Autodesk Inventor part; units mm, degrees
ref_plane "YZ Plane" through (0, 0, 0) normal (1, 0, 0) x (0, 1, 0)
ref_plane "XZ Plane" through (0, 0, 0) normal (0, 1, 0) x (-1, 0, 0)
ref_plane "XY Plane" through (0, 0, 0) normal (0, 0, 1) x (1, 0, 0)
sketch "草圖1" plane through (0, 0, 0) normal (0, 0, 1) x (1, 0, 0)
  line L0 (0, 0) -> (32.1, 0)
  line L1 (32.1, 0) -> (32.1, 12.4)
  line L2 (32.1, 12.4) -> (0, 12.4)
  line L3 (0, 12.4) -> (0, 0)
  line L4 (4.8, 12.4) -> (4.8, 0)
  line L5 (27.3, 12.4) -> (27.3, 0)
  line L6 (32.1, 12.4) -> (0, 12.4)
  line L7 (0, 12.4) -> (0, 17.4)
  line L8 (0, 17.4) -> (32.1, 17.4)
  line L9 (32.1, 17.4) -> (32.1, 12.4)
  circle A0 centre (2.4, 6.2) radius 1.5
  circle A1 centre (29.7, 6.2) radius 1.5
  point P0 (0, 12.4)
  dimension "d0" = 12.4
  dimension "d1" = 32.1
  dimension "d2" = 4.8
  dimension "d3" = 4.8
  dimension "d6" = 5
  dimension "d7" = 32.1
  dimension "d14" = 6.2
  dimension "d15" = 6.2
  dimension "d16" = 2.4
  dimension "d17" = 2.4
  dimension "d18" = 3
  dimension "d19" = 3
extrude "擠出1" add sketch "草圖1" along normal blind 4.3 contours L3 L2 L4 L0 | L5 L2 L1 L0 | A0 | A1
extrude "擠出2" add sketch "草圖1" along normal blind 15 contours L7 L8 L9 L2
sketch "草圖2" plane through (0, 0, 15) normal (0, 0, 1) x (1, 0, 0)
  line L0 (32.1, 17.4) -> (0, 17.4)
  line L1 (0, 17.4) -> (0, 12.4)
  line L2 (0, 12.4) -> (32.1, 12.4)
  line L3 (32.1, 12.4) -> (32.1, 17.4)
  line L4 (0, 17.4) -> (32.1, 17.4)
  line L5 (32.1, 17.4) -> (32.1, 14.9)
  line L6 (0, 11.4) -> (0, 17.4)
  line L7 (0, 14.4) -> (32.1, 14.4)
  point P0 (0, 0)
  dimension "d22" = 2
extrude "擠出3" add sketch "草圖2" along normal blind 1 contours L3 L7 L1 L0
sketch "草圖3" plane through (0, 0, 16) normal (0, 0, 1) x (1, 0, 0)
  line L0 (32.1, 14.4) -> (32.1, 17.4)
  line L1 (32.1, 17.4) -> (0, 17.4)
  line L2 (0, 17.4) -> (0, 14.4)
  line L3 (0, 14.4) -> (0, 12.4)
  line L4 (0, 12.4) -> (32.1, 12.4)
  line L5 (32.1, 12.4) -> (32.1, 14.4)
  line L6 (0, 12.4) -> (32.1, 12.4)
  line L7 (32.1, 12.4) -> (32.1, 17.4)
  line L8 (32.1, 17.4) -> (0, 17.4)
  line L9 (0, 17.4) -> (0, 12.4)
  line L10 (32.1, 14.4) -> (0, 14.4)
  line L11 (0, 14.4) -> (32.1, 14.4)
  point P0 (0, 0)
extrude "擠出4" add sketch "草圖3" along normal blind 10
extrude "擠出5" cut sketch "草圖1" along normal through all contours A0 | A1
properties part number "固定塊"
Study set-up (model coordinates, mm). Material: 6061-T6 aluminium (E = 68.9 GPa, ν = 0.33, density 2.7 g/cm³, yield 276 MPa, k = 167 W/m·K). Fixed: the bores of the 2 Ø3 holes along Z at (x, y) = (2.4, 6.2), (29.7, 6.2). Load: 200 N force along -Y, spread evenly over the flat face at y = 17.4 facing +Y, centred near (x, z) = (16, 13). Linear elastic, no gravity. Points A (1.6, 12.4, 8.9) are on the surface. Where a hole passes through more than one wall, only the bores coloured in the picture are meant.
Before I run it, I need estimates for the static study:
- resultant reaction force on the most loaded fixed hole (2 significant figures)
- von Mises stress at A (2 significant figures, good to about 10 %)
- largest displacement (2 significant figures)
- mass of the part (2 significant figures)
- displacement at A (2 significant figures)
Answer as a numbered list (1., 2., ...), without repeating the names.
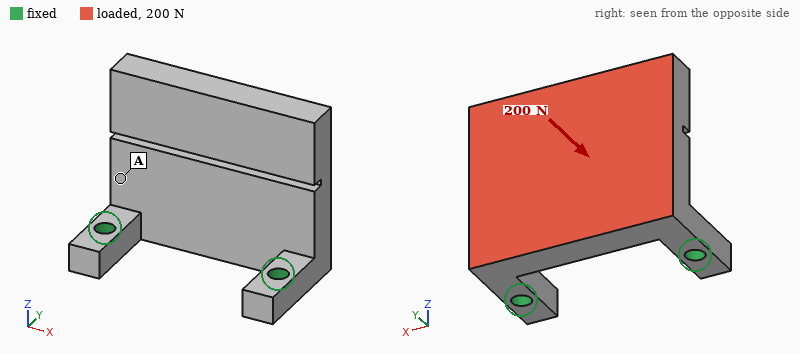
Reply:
1. 100 N
2. 12 MPa
3. 0.10 mm
4. 12 g
5. 0.025 mm
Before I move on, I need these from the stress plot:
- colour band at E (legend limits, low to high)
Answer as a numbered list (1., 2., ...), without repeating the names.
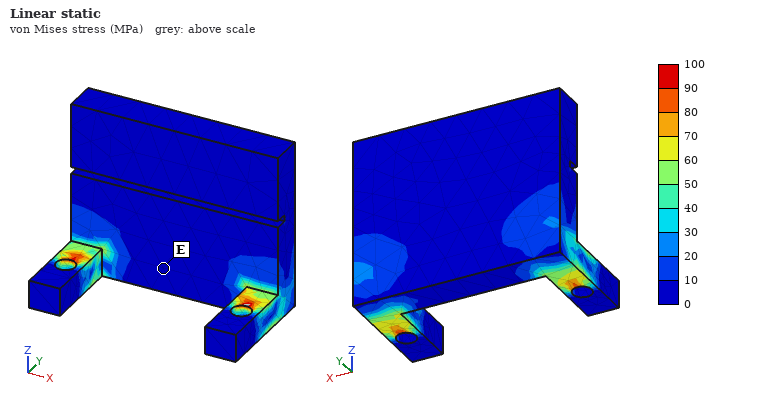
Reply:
1. 0 to 10 MPa
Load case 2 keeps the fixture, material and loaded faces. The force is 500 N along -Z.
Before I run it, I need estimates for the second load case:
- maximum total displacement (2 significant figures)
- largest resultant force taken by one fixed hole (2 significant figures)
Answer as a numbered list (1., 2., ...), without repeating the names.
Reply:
1. 0.15 mm
2. 250 N
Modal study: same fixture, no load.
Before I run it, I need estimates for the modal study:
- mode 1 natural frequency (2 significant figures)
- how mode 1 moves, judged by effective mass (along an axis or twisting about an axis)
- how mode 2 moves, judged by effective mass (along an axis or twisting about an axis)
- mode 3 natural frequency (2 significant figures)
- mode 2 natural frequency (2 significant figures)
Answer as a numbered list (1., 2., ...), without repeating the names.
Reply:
1. 2500 Hz
2. along Y
3. along X
4. 11 kHz
5. 7300 Hz
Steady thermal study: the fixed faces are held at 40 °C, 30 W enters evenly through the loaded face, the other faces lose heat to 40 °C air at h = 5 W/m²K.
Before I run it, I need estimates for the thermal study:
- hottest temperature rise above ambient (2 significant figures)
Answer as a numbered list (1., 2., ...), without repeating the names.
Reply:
1. 45 K
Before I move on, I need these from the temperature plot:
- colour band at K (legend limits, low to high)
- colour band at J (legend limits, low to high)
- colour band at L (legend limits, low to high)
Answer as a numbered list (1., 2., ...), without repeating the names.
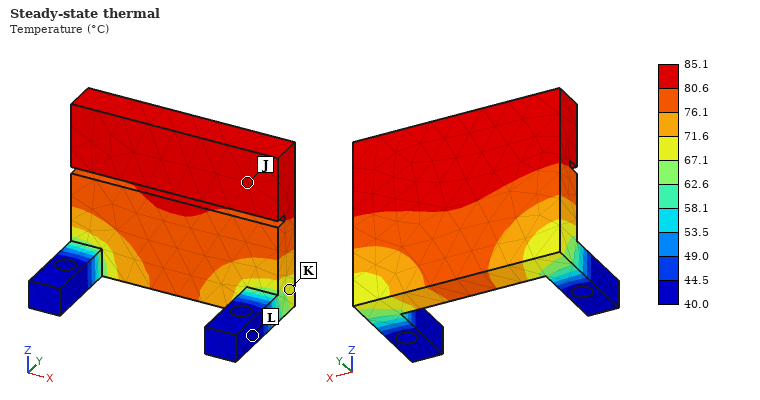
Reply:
1. 67.1 to 71.6 °C
2. 80.6 to 85.1 °C
3. 40.0 to 44.5 °C
